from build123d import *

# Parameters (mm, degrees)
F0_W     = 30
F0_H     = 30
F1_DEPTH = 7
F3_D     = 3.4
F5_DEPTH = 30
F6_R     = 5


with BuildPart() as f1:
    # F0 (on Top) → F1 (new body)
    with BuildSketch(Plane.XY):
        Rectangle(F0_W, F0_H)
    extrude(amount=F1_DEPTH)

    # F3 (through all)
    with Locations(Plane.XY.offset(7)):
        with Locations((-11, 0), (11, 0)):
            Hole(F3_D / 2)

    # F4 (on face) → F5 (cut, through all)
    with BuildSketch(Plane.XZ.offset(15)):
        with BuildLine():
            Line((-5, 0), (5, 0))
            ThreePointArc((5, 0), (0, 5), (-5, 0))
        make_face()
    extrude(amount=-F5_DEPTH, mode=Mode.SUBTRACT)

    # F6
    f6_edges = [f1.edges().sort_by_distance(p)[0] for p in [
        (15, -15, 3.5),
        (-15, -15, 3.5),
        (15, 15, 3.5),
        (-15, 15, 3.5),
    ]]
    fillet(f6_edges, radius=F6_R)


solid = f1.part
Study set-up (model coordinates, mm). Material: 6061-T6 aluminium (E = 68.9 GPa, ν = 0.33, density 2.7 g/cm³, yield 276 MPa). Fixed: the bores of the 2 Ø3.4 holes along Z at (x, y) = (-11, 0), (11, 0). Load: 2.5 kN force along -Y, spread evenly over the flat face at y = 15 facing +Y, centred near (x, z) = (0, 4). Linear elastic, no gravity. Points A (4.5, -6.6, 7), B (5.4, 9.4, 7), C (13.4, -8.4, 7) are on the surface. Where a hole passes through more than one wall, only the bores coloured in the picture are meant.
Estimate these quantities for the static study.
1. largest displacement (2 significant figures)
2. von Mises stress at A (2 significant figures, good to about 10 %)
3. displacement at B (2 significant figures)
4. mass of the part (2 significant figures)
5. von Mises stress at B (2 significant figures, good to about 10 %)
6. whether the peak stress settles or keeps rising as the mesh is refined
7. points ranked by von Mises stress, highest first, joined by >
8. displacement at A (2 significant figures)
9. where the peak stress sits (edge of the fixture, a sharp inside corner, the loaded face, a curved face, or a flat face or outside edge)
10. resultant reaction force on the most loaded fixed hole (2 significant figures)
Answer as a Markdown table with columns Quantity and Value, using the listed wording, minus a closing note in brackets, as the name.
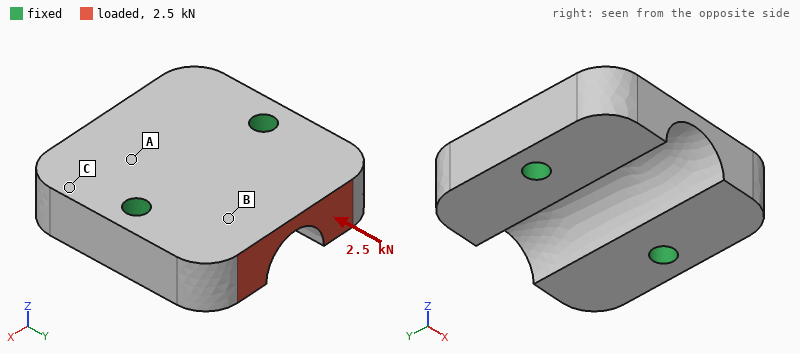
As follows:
| Quantity | Value |
|---|---|
| largest displacement | 10.0 µm |
| von Mises stress at A | 9.9 MPa |
| displacement at B | 5.2 µm |
| mass of the part | 13 g |
| von Mises stress at B | 23 MPa |
| whether the peak stress settles or keeps rising as the mesh is refined | keeps rising |
| points ranked by von Mises stress, highest first, joined by > | B > A > C |
| displacement at A | 2.2 µm |
| where the peak stress sits | edge of the fixture |
| resultant reaction force on the most loaded fixed hole | 1.3 kN |
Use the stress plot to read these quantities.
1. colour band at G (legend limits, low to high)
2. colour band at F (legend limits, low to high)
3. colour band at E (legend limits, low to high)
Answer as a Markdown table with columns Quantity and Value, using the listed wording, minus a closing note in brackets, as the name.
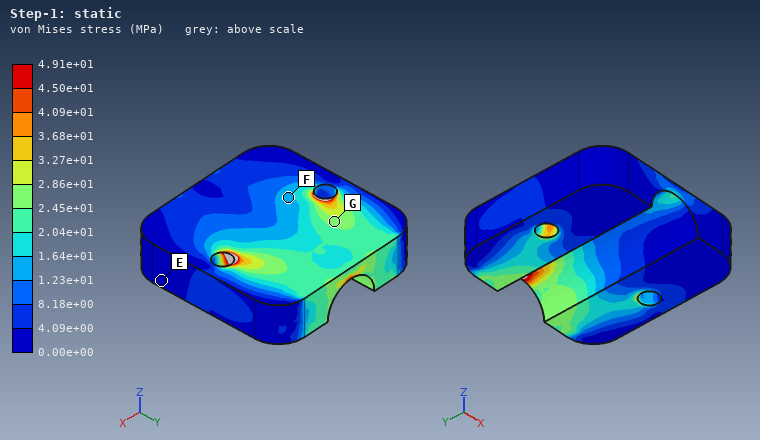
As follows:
| Quantity | Value |
|---|---|
| colour band at G | 2.45e+01 to 2.86e+01 MPa |
| colour band at F | 1.23e+01 to 1.64e+01 MPa |
| colour band at E | 0.00e+00 to 4.09e+00 MPa |
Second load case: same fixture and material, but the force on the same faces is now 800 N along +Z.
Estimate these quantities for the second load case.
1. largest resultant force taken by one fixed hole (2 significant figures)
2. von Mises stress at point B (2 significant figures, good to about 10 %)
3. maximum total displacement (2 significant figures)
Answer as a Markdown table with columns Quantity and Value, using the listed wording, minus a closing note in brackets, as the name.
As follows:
| Quantity | Value |
|---|---|
| largest resultant force taken by one fixed hole | 410 N |
| von Mises stress at point B | 26 MPa |
| maximum total displacement | 34 µm |
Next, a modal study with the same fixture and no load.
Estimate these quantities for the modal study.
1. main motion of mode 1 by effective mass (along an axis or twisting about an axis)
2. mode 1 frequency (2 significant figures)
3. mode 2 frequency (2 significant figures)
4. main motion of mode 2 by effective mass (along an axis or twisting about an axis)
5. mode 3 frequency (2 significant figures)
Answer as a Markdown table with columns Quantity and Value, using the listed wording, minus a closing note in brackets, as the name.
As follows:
| Quantity | Value |
|---|---|
| main motion of mode 1 by effective mass | twisting about X |
| mode 1 frequency | 20 kHz |
| mode 2 frequency | 24 kHz |
| main motion of mode 2 by effective mass | along Z |
| mode 3 frequency | 26 kHz |
